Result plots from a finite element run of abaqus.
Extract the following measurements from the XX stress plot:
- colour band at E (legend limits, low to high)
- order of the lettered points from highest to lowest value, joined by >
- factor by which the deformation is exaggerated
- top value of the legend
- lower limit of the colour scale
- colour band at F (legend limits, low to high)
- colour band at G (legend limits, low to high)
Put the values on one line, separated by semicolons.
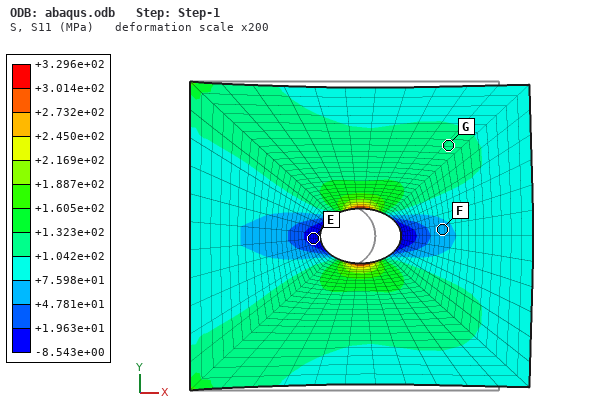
-8.543e+00 to +1.963e+01 MPa; G > F > E; 200; +3.296e+02 MPa; -8.543e+00 MPa; +4.781e+01 to +7.598e+01 MPa; +1.042e+02 to +1.323e+02 MPa
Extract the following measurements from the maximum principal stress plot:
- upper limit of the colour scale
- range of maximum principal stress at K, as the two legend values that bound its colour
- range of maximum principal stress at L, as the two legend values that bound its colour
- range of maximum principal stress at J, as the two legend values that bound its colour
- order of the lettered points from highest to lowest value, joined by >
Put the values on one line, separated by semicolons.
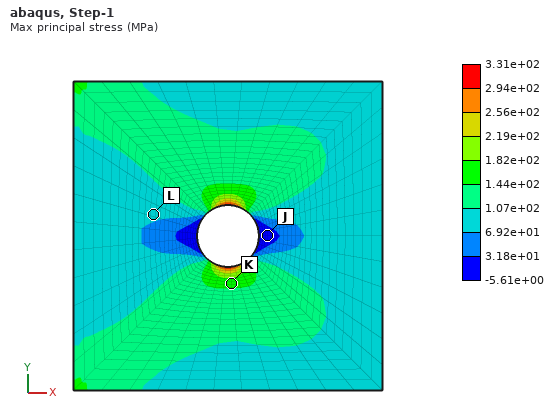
3.31e+02 MPa; 1.44e+02 to 1.82e+02 MPa; 6.92e+01 to 1.07e+02 MPa; -5.61e+00 to 3.18e+01 MPa; K > L > J
